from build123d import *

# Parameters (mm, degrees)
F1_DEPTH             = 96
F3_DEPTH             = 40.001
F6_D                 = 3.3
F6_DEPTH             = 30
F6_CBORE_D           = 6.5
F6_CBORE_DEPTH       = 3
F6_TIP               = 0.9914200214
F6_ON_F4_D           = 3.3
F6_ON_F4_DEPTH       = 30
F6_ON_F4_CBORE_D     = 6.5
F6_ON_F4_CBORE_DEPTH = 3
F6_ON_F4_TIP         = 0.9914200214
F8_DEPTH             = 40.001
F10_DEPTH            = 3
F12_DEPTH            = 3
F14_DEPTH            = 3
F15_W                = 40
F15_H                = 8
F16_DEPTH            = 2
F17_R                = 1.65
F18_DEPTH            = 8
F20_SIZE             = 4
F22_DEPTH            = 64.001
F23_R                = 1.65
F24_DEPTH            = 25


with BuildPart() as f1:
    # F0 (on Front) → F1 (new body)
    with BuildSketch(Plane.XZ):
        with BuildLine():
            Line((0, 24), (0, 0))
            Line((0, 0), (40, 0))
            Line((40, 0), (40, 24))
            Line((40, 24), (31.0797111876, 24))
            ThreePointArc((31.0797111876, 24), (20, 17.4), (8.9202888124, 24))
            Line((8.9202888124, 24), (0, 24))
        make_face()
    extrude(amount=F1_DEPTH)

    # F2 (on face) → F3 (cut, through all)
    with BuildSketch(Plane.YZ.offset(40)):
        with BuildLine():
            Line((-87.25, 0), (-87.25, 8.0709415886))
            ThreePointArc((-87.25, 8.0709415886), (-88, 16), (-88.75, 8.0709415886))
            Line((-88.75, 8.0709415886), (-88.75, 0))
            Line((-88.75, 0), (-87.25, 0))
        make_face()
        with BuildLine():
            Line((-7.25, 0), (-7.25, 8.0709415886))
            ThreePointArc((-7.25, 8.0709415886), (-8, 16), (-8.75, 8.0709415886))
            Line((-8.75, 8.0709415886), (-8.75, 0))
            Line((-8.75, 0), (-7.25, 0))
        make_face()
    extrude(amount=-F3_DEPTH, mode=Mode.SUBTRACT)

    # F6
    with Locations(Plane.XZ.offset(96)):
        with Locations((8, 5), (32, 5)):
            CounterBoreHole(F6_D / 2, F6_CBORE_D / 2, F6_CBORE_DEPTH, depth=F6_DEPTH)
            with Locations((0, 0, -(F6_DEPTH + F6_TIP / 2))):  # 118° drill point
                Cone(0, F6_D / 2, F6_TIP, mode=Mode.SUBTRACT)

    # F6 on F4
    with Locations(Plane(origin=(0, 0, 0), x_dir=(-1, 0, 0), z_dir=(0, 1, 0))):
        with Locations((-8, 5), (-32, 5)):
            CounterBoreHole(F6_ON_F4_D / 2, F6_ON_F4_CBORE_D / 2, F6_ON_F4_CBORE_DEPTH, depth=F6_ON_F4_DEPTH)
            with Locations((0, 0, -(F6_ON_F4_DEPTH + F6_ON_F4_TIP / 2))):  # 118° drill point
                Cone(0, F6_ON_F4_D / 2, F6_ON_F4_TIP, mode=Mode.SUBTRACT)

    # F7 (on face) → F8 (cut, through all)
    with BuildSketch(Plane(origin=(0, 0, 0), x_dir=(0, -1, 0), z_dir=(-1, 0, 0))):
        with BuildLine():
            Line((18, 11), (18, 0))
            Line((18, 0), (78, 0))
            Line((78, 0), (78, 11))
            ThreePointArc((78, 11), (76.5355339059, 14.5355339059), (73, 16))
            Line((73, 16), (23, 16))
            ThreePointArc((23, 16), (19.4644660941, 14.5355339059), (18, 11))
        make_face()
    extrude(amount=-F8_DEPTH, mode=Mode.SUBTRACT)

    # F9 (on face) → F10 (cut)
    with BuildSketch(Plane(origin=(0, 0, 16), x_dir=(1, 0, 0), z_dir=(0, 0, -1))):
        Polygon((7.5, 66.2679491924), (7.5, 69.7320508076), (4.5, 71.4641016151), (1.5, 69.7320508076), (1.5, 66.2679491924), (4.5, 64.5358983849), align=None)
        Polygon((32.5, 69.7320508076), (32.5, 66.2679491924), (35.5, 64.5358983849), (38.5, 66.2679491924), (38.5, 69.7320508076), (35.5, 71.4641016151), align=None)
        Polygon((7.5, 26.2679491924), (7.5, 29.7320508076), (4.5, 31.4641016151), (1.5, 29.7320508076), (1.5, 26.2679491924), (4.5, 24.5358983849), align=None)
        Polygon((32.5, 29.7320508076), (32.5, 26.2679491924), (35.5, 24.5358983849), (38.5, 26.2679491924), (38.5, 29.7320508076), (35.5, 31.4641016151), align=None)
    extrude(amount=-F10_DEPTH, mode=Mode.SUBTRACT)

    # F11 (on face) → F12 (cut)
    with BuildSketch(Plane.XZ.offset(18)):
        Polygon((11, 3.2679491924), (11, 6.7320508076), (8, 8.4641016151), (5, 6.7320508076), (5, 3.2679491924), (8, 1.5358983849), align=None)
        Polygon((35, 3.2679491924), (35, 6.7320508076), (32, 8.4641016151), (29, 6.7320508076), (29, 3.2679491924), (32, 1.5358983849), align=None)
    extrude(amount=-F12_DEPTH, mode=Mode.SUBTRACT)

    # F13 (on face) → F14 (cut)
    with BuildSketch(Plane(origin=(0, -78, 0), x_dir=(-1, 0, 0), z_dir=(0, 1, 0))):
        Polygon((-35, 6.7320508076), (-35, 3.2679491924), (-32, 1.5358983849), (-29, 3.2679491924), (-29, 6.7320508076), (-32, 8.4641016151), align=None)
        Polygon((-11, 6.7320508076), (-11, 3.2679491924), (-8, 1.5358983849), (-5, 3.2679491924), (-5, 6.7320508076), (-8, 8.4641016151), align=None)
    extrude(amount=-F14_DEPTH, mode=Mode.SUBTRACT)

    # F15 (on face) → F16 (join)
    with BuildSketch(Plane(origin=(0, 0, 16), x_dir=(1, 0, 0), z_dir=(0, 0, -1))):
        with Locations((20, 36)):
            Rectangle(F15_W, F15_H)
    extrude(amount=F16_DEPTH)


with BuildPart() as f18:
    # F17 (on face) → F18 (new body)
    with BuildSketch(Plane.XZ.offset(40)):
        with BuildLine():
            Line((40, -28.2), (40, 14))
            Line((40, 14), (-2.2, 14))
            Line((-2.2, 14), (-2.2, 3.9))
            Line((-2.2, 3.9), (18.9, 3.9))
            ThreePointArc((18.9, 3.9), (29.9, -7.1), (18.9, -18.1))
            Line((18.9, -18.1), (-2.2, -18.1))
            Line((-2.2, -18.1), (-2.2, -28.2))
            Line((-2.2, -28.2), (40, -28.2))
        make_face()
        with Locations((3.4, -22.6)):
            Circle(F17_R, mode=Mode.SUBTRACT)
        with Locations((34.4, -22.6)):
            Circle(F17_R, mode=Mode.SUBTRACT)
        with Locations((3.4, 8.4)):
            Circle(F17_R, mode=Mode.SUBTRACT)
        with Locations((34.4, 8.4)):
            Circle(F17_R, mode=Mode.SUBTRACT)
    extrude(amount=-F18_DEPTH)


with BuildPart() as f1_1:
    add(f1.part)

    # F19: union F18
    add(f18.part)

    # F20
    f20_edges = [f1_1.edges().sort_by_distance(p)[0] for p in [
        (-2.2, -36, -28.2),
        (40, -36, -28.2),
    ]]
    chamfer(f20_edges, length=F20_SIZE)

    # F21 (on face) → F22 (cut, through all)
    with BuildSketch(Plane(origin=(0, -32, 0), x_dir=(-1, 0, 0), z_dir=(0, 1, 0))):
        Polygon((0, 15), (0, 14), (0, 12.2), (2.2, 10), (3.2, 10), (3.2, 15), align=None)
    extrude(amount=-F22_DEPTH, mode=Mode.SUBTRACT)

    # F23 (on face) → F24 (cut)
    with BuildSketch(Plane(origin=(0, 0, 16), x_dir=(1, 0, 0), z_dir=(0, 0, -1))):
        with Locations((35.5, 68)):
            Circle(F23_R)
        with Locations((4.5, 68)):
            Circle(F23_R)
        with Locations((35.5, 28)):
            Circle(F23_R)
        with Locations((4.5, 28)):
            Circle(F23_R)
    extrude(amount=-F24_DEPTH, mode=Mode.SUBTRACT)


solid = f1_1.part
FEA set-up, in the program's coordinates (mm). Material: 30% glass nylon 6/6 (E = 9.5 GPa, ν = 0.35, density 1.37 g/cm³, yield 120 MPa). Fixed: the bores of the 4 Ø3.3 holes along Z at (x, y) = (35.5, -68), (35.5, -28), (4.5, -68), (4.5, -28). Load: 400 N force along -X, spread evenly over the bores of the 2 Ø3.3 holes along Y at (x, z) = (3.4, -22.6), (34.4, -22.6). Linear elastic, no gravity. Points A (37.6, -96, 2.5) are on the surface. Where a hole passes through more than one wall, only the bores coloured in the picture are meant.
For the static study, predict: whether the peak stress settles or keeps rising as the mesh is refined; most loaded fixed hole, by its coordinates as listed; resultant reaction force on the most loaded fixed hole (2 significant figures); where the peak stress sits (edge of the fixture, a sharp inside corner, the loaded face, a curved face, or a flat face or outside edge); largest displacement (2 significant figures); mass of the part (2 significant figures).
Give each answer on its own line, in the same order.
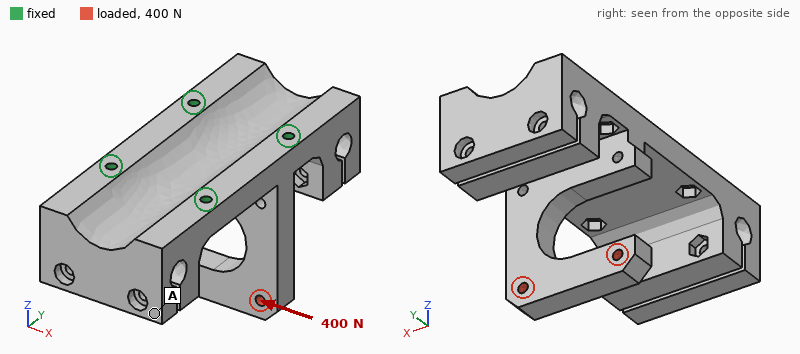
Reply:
keeps rising
(4.5, -28)
640 N
edge of the fixture
0.97 mm
64 g
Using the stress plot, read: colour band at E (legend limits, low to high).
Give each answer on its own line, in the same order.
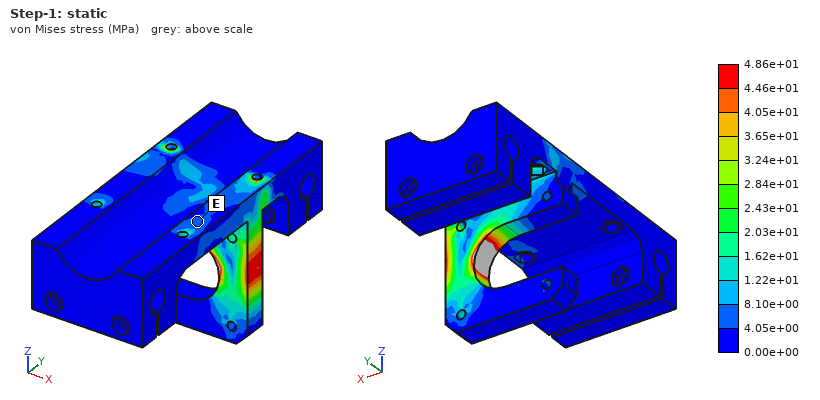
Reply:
4.05e+00 to 8.10e+00 MPa
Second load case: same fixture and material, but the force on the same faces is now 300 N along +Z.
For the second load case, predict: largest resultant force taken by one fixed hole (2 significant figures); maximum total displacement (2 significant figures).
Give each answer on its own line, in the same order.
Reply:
180 N
0.75 mm
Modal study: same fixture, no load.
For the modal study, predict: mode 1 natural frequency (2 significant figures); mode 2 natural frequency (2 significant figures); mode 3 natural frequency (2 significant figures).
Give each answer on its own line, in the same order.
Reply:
890 Hz
1500 Hz
1600 Hz
